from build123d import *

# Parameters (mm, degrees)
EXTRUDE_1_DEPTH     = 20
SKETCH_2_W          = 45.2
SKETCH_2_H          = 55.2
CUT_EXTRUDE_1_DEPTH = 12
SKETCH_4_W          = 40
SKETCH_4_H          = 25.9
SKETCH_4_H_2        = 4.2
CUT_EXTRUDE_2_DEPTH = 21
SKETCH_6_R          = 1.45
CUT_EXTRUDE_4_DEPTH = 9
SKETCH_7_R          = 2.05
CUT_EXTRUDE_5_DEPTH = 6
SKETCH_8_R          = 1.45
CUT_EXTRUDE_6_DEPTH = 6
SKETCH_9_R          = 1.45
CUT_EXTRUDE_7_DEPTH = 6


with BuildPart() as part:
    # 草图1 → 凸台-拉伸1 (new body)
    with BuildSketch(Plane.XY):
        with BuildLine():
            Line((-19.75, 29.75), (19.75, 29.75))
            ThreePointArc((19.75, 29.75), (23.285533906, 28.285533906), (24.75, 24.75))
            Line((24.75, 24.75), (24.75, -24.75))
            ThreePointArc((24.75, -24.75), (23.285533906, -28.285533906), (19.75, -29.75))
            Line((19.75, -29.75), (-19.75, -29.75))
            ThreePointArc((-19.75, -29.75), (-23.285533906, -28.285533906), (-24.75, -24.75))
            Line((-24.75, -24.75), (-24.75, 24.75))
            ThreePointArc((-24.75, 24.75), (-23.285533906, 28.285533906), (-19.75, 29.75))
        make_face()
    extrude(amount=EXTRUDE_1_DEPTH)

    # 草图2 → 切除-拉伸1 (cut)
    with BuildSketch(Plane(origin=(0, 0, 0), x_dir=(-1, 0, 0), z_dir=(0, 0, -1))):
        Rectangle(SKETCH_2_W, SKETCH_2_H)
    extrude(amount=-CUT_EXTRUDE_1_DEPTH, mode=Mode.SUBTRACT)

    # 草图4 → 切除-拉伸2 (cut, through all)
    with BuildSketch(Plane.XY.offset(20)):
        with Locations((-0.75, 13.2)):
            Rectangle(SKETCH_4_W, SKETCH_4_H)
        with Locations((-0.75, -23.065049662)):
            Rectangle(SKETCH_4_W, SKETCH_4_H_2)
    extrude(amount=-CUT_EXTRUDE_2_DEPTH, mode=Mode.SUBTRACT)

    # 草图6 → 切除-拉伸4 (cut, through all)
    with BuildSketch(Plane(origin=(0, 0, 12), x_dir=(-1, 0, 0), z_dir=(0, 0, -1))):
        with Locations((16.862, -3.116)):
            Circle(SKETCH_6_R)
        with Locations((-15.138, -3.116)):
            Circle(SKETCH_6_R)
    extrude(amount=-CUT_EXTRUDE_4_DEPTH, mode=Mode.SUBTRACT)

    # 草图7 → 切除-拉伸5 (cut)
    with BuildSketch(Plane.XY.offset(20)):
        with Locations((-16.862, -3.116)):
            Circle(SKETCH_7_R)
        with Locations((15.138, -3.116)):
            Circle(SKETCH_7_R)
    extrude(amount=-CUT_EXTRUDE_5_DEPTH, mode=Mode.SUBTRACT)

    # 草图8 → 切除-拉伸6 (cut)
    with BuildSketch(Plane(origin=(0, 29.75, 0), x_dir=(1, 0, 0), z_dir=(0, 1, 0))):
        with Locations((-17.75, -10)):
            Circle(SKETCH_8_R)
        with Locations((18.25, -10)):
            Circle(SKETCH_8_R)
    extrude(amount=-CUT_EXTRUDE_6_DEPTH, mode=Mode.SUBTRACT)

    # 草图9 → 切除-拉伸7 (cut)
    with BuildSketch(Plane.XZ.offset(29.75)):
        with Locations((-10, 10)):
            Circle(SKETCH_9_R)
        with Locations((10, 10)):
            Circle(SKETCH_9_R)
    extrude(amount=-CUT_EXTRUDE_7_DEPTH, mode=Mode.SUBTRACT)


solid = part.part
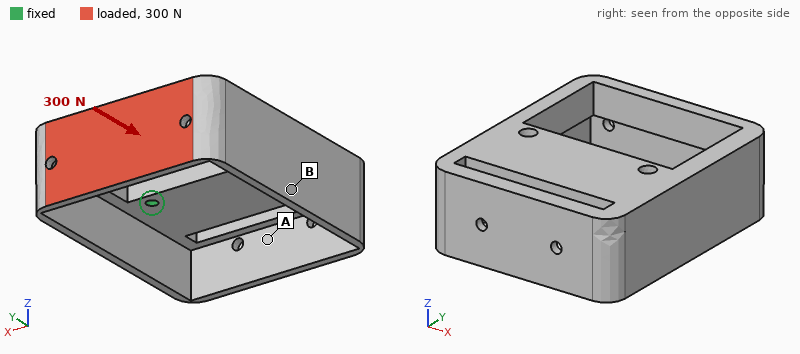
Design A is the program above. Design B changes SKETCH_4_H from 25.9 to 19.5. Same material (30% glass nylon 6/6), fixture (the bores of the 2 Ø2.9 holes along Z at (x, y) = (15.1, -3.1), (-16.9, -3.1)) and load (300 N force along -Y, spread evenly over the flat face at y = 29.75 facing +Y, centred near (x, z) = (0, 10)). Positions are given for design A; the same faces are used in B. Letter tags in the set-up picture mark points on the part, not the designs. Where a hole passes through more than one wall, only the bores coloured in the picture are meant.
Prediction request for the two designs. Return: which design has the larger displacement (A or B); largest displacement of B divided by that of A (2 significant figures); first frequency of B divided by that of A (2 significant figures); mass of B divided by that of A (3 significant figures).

A
0.58
0.98
1.11
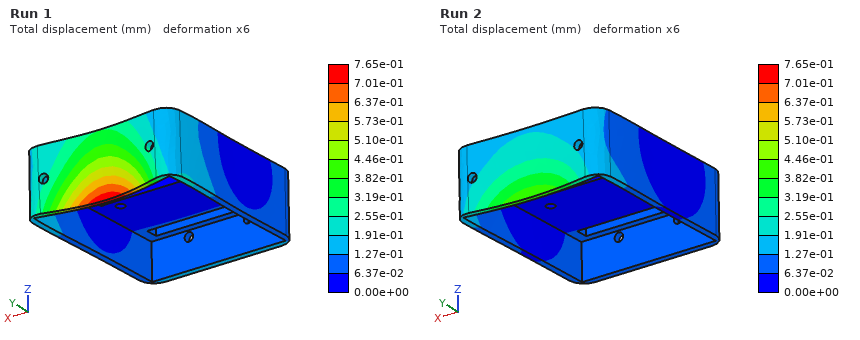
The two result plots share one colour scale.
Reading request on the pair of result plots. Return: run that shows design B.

Run 2
